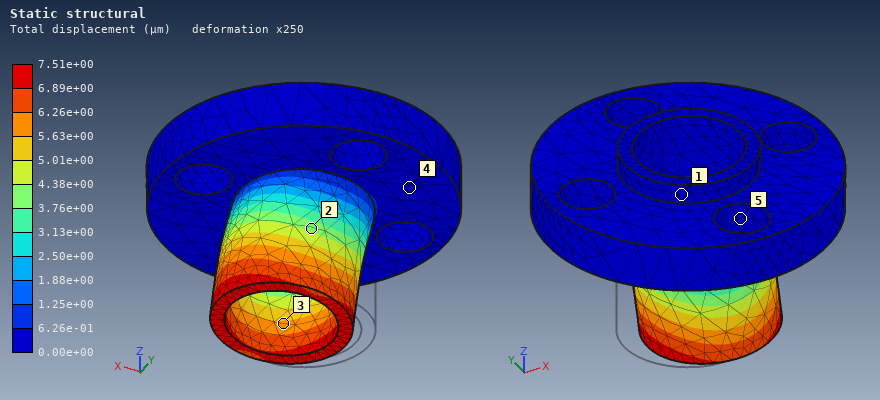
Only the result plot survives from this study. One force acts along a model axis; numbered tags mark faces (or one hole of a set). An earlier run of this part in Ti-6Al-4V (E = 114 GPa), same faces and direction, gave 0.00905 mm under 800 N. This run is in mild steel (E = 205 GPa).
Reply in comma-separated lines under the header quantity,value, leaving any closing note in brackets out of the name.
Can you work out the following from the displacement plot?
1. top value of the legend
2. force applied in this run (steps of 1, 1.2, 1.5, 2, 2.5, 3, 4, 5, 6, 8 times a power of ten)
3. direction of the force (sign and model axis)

quantity,value
top value of the legend,7.51e+00 µm
force applied in this run,1.2 kN
direction of the force,+X
